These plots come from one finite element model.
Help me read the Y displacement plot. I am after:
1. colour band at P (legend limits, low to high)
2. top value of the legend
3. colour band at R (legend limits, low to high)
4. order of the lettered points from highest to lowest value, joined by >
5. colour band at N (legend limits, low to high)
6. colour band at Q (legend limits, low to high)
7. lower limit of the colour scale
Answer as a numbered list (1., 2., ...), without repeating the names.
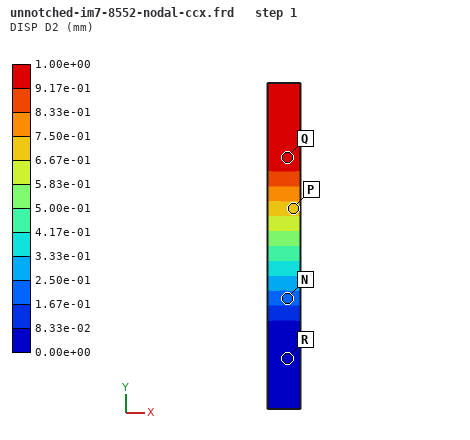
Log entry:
1. 6.67e-01 to 7.50e-01 mm
2. 1.00e+00 mm
3. 0.00e+00 to 8.33e-02 mm
4. Q > P > N > R
5. 1.67e-01 to 2.50e-01 mm
6. 9.17e-01 to 1.00e+00 mm
7. 0.00e+00 mm
